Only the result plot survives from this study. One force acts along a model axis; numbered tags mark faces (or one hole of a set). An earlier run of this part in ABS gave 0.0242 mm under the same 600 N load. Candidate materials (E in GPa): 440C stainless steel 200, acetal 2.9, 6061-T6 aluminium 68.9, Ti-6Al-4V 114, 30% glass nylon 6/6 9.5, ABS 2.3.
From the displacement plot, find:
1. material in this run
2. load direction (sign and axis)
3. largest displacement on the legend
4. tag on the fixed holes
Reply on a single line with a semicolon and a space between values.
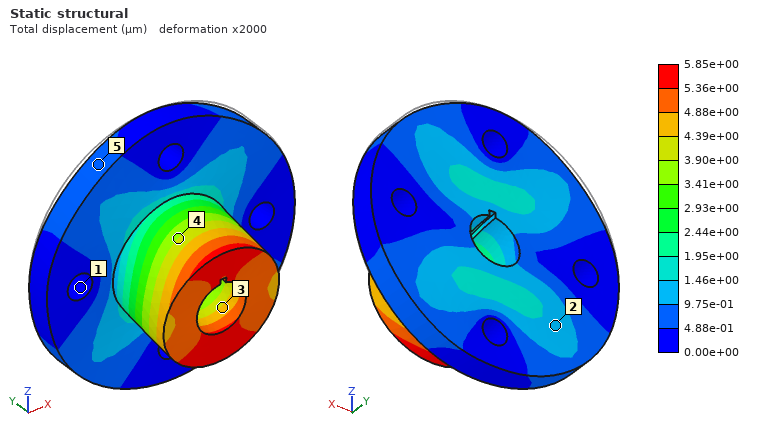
30% glass nylon 6/6; -Z; 5.85e+00 µm; 1
